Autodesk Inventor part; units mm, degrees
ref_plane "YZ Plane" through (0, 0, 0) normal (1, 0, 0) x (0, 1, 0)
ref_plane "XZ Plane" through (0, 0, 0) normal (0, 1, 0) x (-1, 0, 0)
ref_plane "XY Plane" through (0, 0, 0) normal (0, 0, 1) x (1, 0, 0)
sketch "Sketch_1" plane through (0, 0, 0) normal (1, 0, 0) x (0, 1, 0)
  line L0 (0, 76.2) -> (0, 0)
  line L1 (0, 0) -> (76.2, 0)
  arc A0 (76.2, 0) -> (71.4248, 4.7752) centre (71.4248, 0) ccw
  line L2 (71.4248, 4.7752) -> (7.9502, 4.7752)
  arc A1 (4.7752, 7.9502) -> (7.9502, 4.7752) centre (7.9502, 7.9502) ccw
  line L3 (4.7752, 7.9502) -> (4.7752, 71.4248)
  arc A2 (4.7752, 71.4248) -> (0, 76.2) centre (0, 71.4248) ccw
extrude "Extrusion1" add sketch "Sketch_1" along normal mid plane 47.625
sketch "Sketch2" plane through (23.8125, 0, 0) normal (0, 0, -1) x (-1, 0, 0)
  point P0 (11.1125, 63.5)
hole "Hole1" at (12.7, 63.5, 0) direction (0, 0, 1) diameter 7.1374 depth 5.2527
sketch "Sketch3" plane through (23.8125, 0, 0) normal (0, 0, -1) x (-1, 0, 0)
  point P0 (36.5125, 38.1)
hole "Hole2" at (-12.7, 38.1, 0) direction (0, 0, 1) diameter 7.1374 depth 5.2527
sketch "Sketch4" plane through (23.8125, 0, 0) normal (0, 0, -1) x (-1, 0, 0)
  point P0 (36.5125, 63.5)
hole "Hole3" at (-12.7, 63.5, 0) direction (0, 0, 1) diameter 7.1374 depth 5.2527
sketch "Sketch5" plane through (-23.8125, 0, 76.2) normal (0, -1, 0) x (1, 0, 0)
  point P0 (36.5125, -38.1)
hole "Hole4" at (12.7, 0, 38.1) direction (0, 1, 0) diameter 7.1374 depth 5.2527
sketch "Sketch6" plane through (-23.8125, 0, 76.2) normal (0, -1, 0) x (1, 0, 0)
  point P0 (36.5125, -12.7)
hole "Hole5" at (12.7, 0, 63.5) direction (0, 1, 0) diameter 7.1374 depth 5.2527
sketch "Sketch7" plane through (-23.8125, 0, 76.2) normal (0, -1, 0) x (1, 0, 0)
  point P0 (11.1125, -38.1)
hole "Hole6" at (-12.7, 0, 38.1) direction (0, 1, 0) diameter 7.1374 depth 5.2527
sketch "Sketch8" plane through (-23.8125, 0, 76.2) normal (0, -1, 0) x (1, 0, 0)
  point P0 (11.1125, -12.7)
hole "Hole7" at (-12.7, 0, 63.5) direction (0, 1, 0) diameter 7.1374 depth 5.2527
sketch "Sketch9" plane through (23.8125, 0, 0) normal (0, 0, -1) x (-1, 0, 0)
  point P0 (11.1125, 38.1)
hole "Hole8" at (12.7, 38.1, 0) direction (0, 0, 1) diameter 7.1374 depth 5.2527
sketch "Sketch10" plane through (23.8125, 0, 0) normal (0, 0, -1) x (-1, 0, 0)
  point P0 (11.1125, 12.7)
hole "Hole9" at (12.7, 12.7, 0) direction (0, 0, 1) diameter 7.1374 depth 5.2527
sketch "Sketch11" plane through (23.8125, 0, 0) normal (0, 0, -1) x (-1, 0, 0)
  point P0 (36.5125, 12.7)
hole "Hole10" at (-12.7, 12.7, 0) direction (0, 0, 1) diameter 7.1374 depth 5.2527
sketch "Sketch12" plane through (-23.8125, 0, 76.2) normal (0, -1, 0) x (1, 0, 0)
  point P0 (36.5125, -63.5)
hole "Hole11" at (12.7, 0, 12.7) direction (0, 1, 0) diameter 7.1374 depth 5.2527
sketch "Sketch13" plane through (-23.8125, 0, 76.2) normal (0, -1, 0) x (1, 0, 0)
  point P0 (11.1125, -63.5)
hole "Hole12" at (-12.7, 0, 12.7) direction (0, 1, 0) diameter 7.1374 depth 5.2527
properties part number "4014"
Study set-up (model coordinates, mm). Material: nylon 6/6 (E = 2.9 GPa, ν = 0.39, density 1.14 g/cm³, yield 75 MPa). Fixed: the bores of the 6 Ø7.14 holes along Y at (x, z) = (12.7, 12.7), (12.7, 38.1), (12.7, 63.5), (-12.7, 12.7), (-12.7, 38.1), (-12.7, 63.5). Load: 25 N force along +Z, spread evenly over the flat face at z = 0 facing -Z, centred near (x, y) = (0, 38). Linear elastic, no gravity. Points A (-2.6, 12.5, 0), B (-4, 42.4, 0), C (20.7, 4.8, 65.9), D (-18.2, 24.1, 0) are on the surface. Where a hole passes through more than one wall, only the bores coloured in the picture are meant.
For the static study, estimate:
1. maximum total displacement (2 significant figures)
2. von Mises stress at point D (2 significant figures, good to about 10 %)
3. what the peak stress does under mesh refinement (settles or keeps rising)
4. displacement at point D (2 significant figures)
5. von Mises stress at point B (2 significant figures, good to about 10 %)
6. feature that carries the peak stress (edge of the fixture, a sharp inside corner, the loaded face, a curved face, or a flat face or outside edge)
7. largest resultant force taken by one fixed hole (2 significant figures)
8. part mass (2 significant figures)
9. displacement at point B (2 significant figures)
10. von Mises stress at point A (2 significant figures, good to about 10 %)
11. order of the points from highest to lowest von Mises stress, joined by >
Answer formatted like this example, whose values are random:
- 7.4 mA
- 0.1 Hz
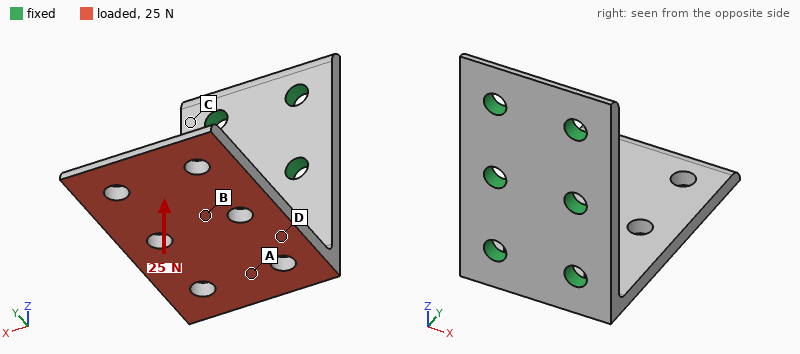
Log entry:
- 1.3 mm
- 2.5 MPa
- keeps rising
- 0.22 mm
- 1.3 MPa
- edge of the fixture
- 13 N
- 35 g
- 0.55 mm
- 4.3 MPa
- A > D > B > C
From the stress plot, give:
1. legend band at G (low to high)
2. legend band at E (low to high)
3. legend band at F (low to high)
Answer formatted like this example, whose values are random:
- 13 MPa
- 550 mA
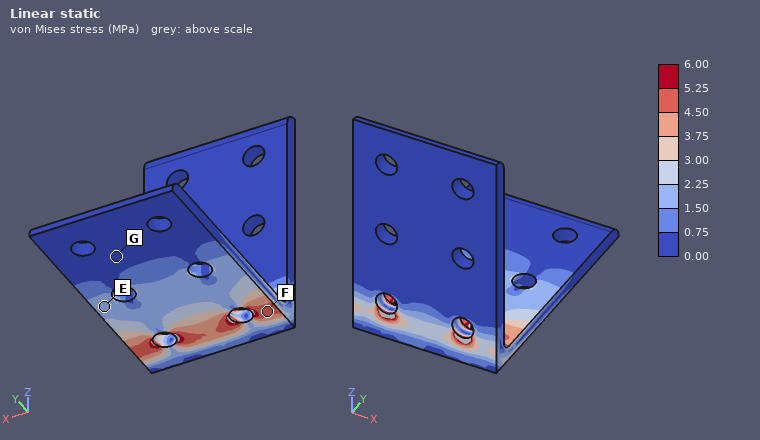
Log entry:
- 0.00 to 0.75 MPa
- 1.50 to 2.25 MPa
- 4.50 to 5.25 MPa
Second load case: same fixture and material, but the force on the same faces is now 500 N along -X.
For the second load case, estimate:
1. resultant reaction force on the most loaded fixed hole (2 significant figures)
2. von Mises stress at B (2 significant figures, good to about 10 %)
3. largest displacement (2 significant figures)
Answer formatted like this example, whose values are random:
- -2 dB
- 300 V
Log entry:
- 670 N
- 5.2 MPa
- 1.3 mm
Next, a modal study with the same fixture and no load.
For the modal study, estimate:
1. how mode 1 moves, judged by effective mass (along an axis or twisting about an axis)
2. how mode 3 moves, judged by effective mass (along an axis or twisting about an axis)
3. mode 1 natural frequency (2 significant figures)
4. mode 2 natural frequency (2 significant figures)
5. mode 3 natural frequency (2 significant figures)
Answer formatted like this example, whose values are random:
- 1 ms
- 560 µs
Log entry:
- along Z
- along X
- 210 Hz
- 690 Hz
- 930 Hz
